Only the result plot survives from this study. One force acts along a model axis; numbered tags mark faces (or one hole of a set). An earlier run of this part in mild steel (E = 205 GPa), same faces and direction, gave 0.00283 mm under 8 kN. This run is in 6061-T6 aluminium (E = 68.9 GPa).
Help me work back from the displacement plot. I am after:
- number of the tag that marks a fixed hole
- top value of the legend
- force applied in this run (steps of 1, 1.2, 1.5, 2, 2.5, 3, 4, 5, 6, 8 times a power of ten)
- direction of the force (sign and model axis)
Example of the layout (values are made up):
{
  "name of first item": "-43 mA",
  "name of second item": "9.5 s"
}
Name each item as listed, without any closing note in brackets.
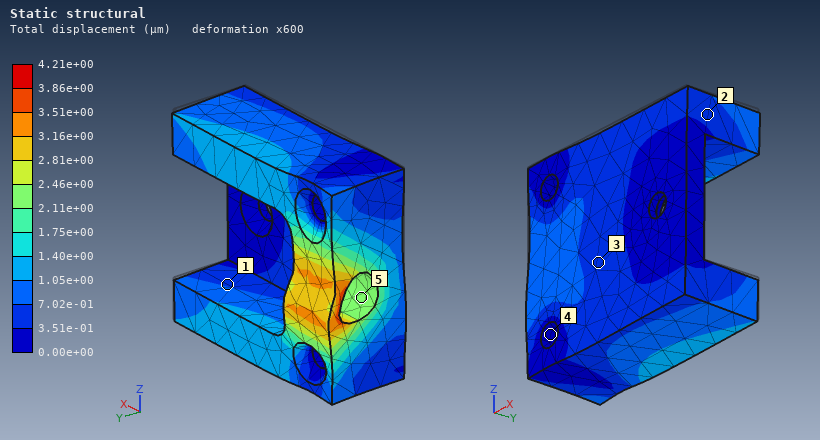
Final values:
{
  "number of the tag that marks a fixed hole": "4",
  "top value of the legend": "4.21e+00 µm",
  "force applied in this run": "4 kN",
  "direction of the force": "-Z"
}
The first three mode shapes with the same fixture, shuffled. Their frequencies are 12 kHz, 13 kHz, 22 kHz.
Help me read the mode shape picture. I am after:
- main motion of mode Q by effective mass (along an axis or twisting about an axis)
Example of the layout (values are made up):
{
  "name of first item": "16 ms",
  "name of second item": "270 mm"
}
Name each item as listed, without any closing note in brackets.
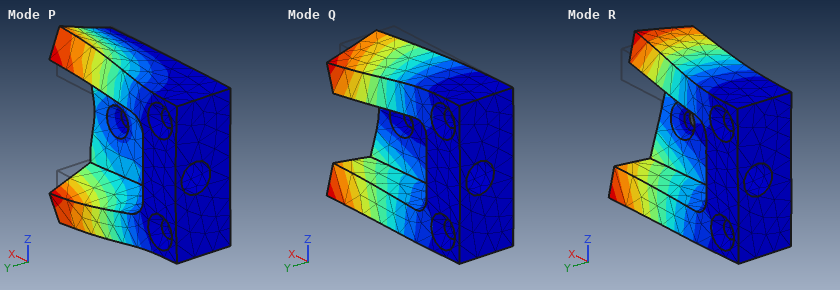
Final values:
{
  "main motion of mode Q by effective mass": "along Y"
}
